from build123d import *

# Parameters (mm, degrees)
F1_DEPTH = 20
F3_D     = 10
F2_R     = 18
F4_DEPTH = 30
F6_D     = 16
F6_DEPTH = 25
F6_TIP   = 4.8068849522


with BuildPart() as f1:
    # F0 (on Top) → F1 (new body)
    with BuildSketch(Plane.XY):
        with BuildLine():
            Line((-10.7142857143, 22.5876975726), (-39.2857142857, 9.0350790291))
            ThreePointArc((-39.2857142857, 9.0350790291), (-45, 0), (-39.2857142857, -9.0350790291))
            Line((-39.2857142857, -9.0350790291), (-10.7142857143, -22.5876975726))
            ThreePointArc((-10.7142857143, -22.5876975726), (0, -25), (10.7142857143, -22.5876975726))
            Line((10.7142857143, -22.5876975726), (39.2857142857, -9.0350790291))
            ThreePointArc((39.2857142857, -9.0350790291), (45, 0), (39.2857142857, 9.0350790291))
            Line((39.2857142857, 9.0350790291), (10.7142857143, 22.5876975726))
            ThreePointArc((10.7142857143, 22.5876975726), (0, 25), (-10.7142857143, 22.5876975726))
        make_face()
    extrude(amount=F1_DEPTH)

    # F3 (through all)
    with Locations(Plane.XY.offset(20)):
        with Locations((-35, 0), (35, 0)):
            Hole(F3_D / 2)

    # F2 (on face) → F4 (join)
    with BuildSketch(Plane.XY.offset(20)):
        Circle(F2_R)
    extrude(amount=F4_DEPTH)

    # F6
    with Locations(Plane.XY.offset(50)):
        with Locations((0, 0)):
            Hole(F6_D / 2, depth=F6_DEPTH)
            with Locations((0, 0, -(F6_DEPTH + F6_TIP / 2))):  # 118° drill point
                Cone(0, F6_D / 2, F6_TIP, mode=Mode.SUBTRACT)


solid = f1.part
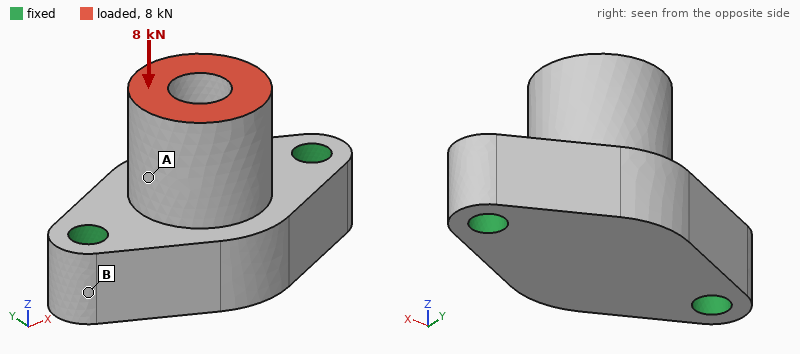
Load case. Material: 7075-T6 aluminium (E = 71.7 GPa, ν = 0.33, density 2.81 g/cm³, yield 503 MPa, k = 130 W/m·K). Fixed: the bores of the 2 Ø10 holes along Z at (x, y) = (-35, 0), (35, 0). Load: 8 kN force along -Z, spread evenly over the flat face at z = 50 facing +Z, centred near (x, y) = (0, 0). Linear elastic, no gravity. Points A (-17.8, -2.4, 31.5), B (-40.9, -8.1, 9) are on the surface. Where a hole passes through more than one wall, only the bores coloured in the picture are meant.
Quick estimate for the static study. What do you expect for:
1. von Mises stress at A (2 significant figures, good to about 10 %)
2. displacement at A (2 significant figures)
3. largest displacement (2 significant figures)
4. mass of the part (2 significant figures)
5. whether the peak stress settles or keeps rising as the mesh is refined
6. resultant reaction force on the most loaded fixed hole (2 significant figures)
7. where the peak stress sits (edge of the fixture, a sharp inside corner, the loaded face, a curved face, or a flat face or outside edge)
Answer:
11 MPa
11 µm
13 µm
230 g
keeps rising
4.1 kN
edge of the fixture
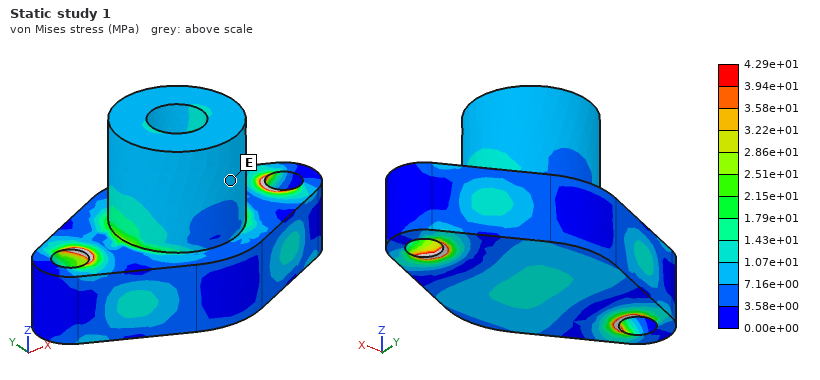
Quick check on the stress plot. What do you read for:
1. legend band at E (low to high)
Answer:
7.16e+00 to 1.07e+01 MPa
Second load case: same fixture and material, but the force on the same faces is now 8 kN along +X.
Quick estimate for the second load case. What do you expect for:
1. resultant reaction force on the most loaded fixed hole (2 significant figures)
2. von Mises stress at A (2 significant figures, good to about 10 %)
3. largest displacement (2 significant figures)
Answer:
6.9 kN
35 MPa
60 µm
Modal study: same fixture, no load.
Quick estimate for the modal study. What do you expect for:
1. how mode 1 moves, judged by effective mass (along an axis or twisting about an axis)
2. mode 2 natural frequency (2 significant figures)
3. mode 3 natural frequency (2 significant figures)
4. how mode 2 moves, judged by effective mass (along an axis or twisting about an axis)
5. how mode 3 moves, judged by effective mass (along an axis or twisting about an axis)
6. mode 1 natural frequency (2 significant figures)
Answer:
along Y
11 kHz
12 kHz
along Z
along X
6100 Hz
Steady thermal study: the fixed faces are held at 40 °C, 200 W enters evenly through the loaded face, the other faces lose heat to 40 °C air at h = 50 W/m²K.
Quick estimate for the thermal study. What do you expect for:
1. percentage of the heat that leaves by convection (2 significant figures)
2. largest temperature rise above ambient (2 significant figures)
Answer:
10 %
84 K
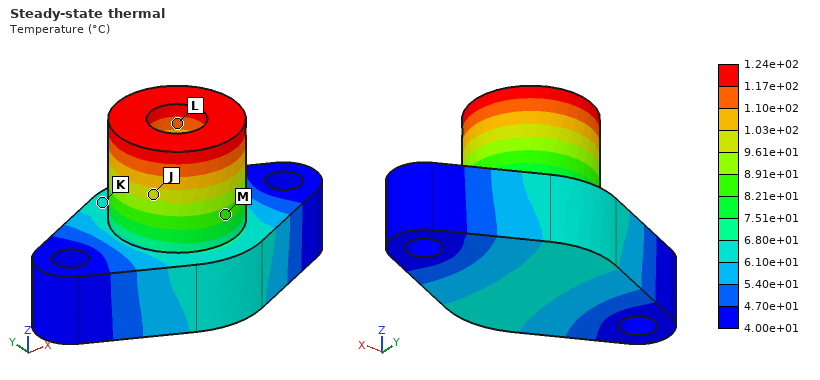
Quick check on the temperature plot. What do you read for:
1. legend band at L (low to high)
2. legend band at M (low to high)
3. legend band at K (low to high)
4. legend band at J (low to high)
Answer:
1.10e+02 to 1.17e+02 °C
8.21e+01 to 8.91e+01 °C
6.10e+01 to 6.80e+01 °C
9.61e+01 to 1.03e+02 °C
